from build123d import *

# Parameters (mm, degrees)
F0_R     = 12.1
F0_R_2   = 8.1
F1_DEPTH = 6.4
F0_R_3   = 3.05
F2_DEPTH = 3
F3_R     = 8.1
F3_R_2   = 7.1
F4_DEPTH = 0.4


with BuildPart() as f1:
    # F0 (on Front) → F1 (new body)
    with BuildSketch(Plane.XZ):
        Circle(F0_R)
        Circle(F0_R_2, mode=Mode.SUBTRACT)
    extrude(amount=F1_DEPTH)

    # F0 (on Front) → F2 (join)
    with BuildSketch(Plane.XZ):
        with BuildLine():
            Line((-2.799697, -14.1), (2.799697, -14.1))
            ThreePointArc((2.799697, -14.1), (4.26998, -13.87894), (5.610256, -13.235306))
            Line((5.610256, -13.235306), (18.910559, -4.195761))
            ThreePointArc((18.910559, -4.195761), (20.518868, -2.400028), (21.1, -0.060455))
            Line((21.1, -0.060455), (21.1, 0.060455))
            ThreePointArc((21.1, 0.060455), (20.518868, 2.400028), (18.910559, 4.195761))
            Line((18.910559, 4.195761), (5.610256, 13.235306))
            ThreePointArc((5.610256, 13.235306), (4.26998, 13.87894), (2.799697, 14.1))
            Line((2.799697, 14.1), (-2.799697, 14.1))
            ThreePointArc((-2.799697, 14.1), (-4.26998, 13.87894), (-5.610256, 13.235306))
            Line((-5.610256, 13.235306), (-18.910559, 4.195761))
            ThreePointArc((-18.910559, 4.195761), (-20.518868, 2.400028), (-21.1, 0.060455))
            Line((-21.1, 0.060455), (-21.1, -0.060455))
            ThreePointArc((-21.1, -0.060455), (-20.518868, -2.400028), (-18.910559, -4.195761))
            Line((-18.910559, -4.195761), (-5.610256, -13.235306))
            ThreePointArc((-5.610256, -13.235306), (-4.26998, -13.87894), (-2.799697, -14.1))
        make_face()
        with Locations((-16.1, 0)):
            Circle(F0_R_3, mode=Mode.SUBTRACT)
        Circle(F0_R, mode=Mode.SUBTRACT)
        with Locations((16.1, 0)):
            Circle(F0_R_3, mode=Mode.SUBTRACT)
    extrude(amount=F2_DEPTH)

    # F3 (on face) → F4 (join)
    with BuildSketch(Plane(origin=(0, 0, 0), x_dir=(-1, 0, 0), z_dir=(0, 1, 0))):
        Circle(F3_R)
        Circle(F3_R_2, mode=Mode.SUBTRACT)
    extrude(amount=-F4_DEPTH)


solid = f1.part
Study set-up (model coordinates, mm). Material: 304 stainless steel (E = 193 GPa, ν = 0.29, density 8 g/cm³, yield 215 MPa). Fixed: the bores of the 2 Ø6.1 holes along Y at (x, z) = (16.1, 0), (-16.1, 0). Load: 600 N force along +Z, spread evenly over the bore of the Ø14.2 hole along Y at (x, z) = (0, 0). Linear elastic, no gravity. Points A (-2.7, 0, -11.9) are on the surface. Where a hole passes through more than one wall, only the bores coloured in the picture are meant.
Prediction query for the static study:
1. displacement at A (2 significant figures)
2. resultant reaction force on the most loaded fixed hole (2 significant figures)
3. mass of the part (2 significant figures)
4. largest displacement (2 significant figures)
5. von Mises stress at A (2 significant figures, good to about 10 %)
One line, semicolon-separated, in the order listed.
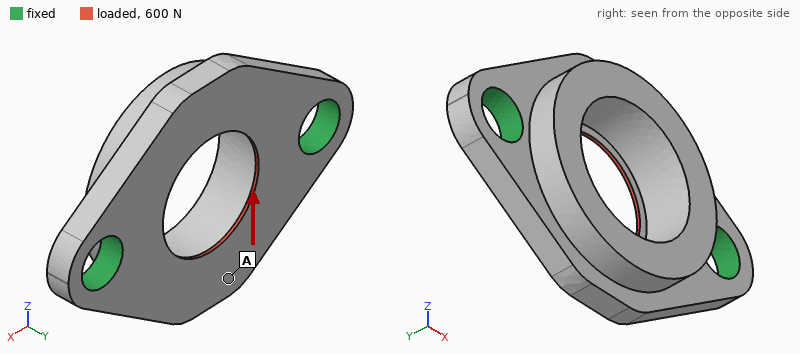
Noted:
2.2 µm; 300 N; 20 g; 2.7 µm; 7.4 MPa
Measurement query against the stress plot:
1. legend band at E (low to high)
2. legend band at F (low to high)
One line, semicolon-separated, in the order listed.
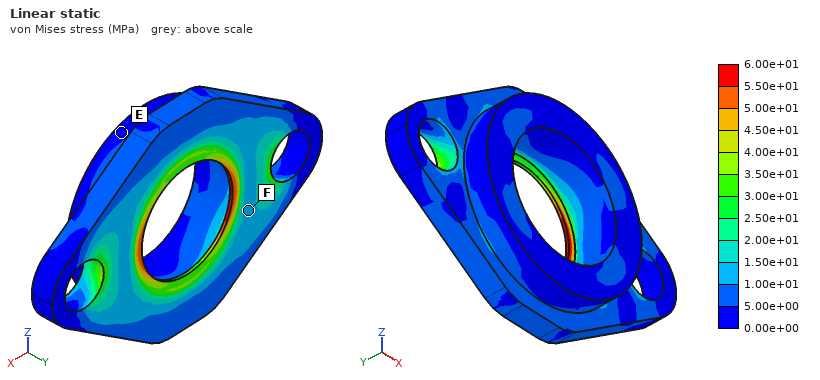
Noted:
0.00e+00 to 5.00e+00 MPa; 1.00e+01 to 1.50e+01 MPa
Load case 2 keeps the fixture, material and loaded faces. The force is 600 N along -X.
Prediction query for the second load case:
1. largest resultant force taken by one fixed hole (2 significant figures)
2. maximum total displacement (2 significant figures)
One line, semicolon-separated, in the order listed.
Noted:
300 N; 1.2 µm
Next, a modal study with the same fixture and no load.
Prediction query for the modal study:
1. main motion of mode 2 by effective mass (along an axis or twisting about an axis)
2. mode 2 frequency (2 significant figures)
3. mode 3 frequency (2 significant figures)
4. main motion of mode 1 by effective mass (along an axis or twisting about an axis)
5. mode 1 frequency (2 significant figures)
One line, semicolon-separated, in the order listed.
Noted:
along Y; 15 kHz; 35 kHz; twisting about X; 12 kHz
